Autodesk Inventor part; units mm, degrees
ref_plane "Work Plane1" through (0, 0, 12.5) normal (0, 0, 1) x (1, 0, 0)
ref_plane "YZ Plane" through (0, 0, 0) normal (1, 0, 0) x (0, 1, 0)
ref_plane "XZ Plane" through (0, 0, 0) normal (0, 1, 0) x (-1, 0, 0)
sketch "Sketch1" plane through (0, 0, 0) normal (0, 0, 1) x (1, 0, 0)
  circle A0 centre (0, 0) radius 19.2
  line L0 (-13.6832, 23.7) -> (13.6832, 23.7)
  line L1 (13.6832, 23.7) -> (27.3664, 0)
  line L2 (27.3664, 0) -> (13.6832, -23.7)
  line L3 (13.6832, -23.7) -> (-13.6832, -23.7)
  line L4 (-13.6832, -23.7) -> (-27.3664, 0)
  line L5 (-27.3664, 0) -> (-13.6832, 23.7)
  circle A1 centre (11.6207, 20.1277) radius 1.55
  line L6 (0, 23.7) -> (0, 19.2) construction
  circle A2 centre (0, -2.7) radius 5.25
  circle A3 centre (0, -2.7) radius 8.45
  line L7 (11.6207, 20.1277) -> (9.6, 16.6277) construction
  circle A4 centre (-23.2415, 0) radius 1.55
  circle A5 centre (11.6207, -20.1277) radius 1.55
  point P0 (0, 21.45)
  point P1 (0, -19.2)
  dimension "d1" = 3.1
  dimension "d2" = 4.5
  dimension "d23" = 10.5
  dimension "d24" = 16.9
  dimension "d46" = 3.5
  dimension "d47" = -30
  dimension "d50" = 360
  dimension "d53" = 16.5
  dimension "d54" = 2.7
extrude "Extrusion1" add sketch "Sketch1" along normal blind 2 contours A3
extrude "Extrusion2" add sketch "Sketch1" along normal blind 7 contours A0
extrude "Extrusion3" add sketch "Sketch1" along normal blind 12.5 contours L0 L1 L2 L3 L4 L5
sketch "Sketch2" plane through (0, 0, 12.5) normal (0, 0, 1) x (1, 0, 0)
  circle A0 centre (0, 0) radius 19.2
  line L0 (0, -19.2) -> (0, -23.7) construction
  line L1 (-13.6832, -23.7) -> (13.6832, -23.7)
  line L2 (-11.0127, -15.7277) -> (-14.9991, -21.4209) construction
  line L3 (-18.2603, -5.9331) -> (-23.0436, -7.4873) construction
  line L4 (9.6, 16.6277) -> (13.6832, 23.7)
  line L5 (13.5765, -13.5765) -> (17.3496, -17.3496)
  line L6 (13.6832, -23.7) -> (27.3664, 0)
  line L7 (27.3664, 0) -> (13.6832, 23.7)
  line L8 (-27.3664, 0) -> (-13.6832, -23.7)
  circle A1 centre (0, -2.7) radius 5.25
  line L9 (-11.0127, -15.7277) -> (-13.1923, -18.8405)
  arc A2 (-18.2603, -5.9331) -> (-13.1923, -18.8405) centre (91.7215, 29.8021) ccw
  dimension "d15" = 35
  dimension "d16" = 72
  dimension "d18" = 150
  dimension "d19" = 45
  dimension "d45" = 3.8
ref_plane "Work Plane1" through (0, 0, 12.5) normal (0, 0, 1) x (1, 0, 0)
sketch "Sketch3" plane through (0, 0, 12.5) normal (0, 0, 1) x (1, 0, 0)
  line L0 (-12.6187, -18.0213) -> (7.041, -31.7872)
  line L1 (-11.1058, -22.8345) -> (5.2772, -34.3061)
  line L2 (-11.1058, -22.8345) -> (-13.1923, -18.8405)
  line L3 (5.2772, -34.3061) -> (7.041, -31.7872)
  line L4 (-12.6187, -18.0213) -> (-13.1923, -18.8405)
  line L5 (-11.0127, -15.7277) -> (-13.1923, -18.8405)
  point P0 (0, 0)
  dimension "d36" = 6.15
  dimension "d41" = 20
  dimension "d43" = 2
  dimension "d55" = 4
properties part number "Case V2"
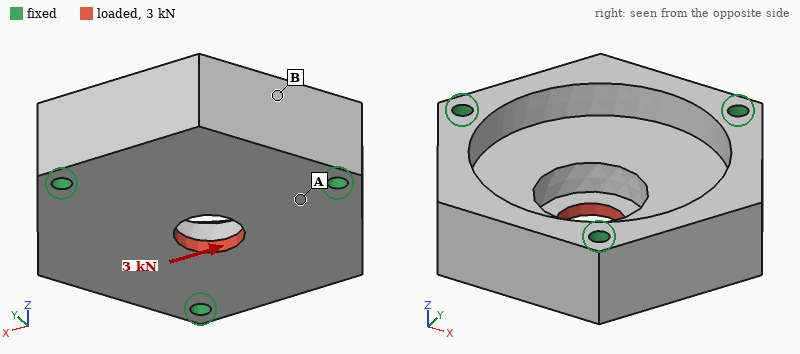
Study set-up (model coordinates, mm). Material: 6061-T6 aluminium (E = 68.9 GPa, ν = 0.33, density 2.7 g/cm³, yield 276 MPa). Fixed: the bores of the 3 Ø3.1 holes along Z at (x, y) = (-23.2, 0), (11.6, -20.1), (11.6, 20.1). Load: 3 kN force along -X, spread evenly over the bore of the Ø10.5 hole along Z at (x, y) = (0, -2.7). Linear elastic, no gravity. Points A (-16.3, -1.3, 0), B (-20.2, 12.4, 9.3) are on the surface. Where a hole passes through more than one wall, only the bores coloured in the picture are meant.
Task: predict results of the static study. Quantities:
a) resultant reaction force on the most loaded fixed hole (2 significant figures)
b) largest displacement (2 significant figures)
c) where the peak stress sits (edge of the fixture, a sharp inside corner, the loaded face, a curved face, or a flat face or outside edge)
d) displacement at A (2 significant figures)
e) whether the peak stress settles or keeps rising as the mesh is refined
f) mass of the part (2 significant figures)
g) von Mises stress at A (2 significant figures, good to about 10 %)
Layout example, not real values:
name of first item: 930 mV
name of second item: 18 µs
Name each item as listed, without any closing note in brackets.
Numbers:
resultant reaction force on the most loaded fixed hole: 1.1 kN
largest displacement: 11 µm
where the peak stress sits: a sharp inside corner
displacement at A: 1.8 µm
whether the peak stress settles or keeps rising as the mesh is refined: keeps rising
mass of the part: 44 g
von Mises stress at A: 23 MPa
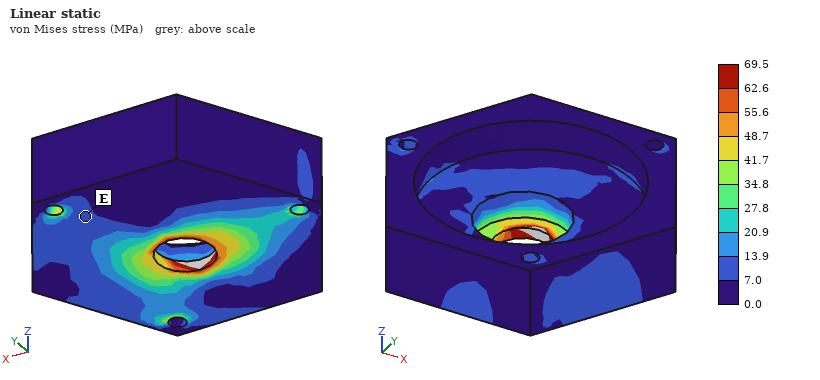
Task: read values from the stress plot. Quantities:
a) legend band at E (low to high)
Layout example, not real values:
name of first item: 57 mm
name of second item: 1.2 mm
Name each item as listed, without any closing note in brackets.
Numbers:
legend band at E: 7.0 to 13.9 MPa
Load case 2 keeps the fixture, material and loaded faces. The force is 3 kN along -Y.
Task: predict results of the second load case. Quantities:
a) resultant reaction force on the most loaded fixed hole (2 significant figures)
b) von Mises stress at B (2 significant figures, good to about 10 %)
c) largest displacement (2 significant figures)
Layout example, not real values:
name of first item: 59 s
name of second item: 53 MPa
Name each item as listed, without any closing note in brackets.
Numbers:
resultant reaction force on the most loaded fixed hole: 1.1 kN
von Mises stress at B: 7.3 MPa
largest displacement: 10 µm
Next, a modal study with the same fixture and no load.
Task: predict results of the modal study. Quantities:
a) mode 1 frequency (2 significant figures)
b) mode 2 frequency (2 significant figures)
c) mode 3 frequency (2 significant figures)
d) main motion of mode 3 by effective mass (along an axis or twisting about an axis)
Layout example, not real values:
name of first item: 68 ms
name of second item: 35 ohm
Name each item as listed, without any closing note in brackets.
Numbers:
mode 1 frequency: 18 kHz
mode 2 frequency: 18 kHz
mode 3 frequency: 19 kHz
main motion of mode 3 by effective mass: along Z
